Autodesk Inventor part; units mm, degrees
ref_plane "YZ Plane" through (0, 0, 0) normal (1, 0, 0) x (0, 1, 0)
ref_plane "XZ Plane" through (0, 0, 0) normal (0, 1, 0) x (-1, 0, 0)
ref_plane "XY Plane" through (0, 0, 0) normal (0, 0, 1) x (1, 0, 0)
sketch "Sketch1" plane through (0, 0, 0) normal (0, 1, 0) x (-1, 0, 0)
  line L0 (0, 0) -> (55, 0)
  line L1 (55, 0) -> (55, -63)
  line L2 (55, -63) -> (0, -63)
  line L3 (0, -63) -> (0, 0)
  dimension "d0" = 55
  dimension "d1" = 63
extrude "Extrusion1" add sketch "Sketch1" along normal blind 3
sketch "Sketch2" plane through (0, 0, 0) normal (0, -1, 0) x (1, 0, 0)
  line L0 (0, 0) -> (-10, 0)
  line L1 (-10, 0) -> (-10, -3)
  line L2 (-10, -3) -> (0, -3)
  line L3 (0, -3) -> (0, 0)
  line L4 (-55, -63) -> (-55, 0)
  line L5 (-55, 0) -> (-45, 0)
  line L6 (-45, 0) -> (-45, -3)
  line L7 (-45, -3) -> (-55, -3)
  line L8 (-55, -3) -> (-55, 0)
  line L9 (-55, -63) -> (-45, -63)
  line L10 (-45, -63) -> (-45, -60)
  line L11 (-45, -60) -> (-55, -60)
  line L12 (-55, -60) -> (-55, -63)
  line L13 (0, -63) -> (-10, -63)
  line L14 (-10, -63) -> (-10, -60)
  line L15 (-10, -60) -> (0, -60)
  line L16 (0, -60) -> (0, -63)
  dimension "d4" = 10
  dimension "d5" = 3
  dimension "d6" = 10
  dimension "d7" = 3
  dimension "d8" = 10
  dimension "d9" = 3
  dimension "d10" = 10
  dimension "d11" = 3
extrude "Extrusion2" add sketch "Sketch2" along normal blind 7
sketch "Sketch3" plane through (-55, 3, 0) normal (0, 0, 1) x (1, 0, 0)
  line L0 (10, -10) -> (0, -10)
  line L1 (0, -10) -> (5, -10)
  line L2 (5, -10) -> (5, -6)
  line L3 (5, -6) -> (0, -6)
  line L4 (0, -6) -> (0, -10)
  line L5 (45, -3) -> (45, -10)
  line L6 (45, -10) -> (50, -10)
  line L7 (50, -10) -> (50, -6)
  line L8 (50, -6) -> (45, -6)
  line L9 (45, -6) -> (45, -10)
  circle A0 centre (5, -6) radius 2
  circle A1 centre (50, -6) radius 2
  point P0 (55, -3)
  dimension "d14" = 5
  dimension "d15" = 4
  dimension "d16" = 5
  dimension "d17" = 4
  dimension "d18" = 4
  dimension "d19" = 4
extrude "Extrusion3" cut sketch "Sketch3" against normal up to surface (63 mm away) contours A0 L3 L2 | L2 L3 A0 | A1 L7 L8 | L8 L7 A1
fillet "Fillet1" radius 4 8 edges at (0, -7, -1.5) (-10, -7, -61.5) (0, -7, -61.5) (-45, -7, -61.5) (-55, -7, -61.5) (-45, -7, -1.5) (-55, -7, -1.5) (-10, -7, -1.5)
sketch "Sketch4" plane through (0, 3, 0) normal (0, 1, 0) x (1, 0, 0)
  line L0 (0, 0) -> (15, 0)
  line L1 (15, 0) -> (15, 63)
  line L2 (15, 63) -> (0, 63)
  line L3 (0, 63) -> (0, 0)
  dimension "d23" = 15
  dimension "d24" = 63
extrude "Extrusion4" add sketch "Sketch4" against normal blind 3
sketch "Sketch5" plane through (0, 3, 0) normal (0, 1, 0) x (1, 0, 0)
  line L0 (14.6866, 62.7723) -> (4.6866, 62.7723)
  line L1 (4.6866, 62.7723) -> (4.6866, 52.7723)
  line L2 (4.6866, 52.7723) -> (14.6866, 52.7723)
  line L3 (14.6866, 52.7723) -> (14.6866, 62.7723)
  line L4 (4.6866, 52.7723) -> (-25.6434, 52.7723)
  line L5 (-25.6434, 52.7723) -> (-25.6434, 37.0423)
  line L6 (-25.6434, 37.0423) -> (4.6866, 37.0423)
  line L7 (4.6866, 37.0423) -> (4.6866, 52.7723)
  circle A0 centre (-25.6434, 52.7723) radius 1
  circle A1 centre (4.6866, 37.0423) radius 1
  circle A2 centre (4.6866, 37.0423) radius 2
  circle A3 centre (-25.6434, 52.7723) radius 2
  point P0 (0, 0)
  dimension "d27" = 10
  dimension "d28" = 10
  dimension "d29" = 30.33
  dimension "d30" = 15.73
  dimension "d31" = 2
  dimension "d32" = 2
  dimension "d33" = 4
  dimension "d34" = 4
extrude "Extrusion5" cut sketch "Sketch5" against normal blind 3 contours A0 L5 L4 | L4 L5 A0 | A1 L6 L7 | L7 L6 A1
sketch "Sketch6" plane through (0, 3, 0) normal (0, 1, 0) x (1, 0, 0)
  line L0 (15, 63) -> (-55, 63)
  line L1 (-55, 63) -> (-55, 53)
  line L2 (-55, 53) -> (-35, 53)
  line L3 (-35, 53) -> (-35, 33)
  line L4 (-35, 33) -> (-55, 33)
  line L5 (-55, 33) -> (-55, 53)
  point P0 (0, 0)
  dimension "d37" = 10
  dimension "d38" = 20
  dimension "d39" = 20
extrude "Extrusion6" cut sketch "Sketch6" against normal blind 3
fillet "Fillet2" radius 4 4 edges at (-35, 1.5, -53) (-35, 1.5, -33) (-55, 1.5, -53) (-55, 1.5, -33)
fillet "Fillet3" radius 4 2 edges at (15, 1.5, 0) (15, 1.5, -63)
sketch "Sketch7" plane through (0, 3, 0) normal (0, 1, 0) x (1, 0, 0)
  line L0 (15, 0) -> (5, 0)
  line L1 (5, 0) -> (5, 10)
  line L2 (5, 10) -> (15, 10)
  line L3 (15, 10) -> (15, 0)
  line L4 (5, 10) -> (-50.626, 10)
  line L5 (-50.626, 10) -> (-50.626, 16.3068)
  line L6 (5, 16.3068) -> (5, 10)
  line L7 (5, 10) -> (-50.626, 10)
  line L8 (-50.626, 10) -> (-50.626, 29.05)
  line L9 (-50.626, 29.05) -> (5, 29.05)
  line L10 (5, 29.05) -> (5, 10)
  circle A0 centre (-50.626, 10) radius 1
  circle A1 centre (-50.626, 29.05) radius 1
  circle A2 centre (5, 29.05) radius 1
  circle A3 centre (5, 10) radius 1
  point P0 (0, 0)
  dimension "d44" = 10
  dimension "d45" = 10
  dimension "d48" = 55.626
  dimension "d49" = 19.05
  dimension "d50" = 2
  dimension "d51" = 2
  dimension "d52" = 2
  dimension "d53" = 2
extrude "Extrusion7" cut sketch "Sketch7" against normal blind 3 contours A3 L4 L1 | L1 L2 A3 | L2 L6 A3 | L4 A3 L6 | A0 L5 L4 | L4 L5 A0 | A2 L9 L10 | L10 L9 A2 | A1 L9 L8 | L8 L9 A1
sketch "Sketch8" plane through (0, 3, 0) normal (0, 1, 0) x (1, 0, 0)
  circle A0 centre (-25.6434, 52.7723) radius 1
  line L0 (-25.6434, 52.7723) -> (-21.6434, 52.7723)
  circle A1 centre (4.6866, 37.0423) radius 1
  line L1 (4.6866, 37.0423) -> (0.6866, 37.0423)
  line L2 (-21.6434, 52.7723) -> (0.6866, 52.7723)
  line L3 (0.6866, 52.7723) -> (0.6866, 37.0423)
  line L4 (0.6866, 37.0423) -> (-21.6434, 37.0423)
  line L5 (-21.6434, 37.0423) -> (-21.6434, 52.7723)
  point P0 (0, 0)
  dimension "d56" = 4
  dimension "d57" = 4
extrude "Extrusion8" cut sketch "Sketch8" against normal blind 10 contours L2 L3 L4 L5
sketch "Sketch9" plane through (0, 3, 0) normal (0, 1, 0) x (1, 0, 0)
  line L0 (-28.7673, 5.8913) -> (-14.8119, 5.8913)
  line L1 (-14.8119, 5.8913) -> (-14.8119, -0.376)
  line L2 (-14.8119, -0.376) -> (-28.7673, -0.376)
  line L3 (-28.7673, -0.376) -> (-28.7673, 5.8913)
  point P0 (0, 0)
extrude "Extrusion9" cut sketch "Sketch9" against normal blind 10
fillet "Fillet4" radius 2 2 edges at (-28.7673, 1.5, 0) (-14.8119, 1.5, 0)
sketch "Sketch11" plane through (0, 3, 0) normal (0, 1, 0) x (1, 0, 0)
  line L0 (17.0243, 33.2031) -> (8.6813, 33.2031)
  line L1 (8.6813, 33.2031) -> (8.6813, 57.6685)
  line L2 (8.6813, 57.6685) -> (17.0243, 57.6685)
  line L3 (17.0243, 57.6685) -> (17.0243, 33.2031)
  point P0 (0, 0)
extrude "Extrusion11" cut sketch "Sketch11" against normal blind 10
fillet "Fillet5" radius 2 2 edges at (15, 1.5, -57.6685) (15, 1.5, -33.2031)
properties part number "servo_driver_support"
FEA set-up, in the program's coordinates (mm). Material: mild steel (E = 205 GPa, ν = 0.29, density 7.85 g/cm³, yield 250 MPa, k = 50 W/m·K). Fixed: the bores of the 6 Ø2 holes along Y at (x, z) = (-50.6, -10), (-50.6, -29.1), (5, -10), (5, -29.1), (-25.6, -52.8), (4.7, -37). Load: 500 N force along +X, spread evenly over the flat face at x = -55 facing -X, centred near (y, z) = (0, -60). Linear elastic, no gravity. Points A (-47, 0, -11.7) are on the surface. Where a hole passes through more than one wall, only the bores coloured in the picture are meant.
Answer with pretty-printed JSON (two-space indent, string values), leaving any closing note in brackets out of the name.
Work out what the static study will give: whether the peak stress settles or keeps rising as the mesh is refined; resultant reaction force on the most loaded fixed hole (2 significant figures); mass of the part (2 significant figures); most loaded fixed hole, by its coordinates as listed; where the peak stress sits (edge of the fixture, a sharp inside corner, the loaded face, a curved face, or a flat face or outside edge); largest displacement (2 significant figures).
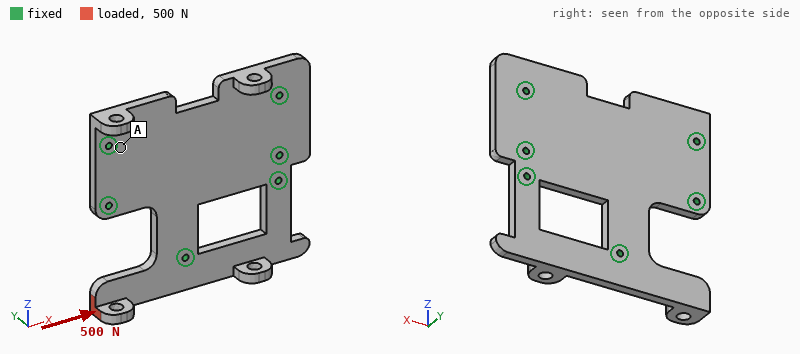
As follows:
{
  "whether the peak stress settles or keeps rising as the mesh is refined": "keeps rising",
  "resultant reaction force on the most loaded fixed hole": "550 N",
  "mass of the part": "85 g",
  "most loaded fixed hole, by its coordinates as listed": "(-25.6, -52.8)",
  "where the peak stress sits": "edge of the fixture",
  "largest displacement": "44 µm"
}
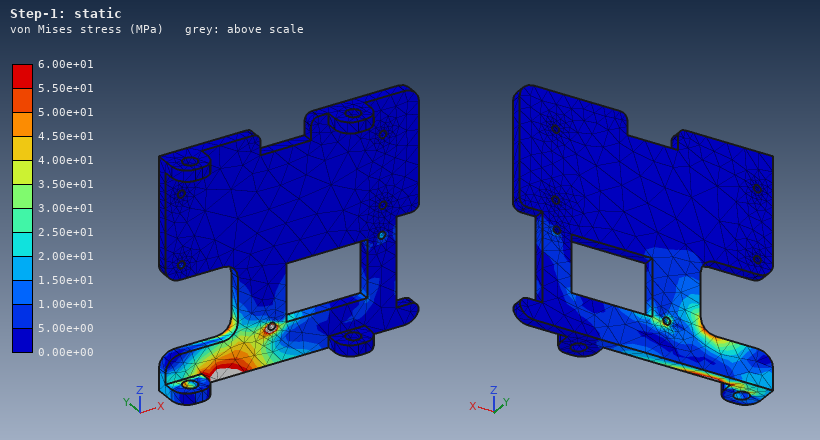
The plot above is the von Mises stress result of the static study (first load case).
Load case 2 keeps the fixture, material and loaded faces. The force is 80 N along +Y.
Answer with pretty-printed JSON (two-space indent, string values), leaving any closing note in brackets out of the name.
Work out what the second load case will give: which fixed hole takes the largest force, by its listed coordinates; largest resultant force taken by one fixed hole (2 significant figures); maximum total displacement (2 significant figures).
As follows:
{
  "which fixed hole takes the largest force, by its listed coordinates": "(-25.6, -52.8)",
  "largest resultant force taken by one fixed hole": "99 N",
  "maximum total displacement": "0.13 mm"
}
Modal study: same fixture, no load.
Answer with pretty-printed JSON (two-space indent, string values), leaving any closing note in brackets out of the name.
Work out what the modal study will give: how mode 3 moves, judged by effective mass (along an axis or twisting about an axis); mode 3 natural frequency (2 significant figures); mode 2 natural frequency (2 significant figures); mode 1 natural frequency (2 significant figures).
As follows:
{
  "how mode 3 moves, judged by effective mass": "along Y",
  "mode 3 natural frequency": "4900 Hz",
  "mode 2 natural frequency": "3400 Hz",
  "mode 1 natural frequency": "2600 Hz"
}
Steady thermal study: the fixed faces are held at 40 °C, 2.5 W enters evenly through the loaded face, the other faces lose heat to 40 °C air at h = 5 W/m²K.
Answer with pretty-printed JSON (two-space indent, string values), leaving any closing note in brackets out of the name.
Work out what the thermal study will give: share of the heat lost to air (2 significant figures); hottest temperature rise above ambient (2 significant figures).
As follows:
{
  "share of the heat lost to air": "5.7 %",
  "hottest temperature rise above ambient": "45 K"
}
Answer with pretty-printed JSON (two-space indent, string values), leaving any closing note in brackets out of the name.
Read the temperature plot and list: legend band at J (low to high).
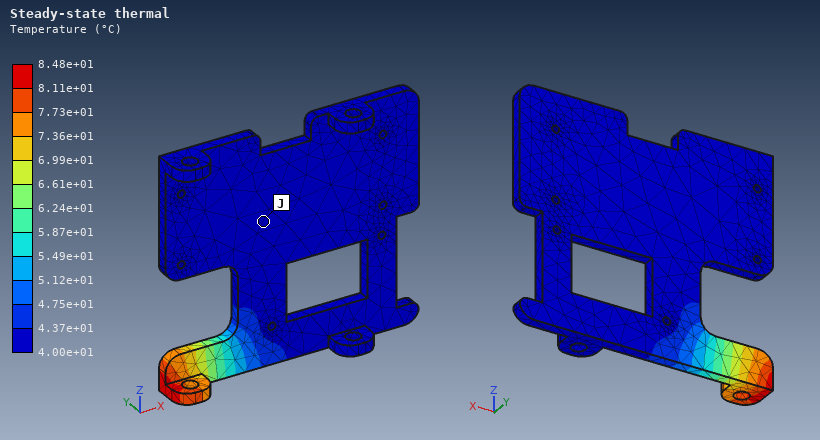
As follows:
{
  "legend band at J": "4.00e+01 to 4.37e+01 °C"
}
